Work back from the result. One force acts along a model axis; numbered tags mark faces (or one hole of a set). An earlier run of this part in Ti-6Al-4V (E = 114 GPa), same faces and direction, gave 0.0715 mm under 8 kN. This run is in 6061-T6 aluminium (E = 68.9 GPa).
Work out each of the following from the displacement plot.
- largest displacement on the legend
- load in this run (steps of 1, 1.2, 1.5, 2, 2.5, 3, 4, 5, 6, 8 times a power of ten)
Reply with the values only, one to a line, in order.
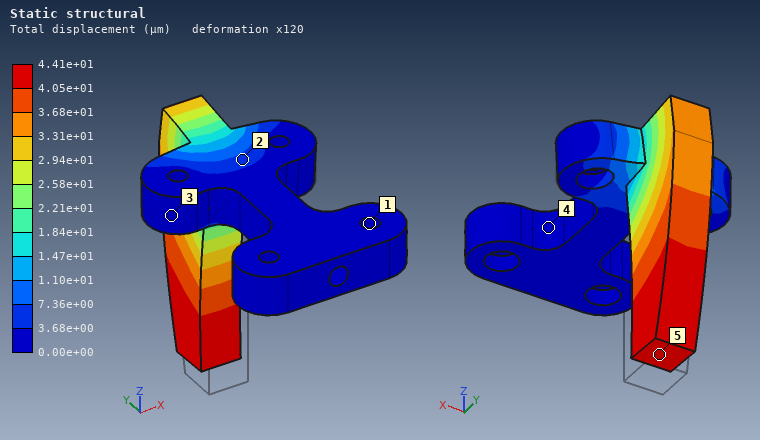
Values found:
4.41e+01 µm
3 kN
